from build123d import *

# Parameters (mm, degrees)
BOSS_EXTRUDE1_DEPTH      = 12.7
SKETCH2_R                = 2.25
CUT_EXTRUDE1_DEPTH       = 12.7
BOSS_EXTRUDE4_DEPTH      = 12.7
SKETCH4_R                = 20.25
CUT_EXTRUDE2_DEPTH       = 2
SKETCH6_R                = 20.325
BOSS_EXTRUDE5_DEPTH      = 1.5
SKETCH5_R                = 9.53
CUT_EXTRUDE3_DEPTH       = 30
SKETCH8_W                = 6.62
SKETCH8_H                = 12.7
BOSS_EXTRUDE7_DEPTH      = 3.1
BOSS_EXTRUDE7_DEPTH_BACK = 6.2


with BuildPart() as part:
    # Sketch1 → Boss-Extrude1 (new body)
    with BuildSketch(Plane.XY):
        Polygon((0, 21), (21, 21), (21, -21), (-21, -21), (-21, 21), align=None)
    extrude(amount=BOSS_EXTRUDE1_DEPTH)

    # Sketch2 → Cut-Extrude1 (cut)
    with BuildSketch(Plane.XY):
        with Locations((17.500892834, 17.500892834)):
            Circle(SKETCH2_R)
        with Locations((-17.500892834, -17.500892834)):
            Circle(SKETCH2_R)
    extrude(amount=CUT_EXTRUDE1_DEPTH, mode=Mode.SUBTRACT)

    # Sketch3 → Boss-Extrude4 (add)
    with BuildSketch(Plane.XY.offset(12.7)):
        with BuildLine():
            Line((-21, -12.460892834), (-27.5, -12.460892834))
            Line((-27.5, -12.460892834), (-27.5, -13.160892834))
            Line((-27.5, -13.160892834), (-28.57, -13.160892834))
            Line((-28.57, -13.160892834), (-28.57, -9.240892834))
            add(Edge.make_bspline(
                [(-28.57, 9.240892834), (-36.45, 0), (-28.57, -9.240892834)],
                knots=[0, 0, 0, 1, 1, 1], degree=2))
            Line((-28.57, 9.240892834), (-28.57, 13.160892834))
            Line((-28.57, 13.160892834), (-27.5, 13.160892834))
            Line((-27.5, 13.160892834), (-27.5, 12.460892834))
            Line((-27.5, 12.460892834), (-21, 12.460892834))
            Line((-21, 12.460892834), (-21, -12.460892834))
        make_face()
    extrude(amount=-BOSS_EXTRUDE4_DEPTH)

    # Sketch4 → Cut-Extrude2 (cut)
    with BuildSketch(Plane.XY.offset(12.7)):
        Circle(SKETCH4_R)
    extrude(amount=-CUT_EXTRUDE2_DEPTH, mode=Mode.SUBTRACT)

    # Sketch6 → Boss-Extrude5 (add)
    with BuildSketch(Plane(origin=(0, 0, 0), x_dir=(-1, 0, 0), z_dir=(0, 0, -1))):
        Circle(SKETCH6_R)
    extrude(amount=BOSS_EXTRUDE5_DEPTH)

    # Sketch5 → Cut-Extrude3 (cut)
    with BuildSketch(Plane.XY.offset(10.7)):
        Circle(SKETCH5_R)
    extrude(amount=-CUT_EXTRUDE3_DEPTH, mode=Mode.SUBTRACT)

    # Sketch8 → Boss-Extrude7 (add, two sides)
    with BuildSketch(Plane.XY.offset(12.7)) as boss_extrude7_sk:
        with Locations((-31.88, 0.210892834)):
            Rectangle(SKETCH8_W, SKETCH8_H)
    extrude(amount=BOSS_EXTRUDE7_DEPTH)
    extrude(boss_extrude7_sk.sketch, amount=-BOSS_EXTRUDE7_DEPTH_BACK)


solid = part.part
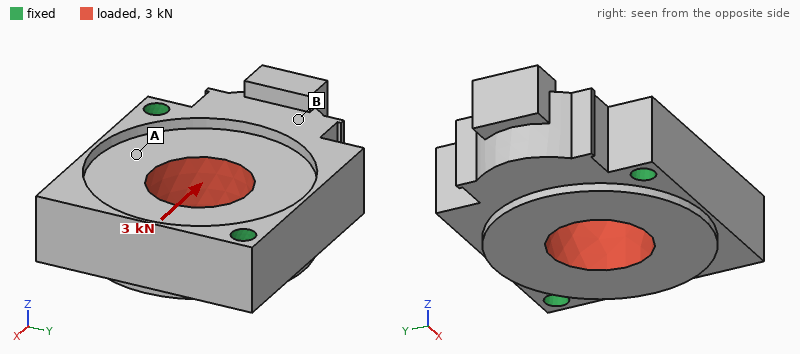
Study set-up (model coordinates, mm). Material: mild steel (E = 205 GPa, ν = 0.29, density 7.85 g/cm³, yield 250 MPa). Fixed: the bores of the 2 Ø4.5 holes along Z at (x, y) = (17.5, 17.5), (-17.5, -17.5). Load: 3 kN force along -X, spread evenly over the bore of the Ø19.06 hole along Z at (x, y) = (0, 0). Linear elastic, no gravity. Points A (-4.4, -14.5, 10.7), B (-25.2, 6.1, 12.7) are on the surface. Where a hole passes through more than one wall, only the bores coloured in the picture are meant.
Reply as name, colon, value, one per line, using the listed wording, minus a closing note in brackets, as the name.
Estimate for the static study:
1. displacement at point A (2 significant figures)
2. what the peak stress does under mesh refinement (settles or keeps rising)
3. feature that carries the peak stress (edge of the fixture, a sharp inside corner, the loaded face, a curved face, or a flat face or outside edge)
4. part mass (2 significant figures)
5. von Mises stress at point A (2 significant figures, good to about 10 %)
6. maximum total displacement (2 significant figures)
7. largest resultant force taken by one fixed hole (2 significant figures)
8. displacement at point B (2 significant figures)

displacement at point A: 0.62 µm
what the peak stress does under mesh refinement: keeps rising
feature that carries the peak stress: edge of the fixture
part mass: 170 g
von Mises stress at point A: 9.4 MPa
maximum total displacement: 1.7 µm
largest resultant force taken by one fixed hole: 1.5 kN
displacement at point B: 1.1 µm
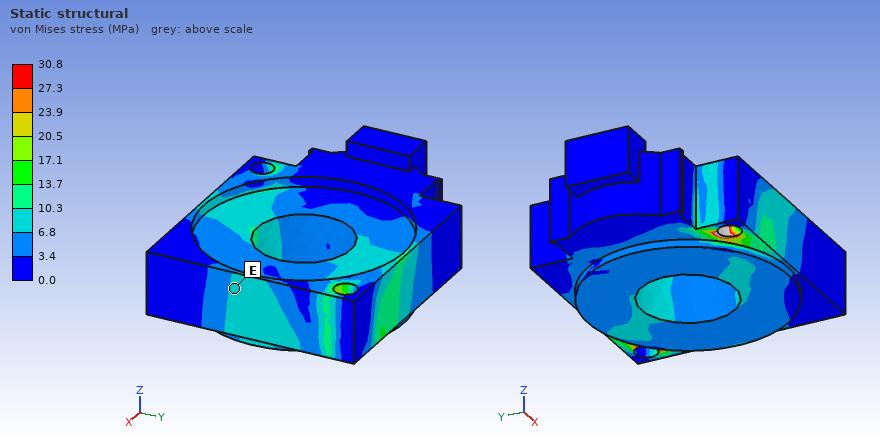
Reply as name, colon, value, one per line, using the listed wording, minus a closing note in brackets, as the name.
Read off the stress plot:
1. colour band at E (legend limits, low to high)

colour band at E: 6.8 to 10.3 MPa
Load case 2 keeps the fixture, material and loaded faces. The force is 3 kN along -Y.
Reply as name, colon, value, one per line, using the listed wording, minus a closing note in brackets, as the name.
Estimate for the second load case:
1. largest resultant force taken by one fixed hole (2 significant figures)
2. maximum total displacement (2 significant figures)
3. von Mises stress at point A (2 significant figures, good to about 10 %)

largest resultant force taken by one fixed hole: 1.5 kN
maximum total displacement: 1.7 µm
von Mises stress at point A: 3.9 MPa
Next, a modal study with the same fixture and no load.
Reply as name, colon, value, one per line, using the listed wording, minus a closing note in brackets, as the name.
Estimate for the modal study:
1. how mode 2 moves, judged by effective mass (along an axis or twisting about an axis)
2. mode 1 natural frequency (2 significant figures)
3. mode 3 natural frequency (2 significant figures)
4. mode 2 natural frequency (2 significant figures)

how mode 2 moves, judged by effective mass: along Z
mode 1 natural frequency: 7600 Hz
mode 3 natural frequency: 17 kHz
mode 2 natural frequency: 11 kHz
